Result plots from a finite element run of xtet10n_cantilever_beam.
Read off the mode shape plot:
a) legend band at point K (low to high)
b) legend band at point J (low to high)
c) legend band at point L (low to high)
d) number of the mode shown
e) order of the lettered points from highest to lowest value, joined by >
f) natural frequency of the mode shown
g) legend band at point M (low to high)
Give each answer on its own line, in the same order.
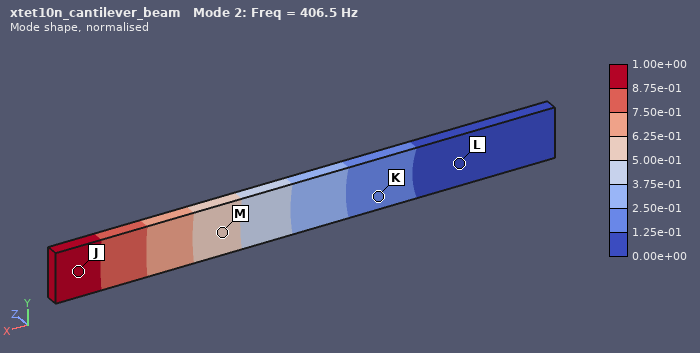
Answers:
1.25e-01 to 2.50e-01
8.75e-01 to 1.00e+00
0.00e+00 to 1.25e-01
2
J > M > K > L
406.5 Hz
5.00e-01 to 6.25e-01
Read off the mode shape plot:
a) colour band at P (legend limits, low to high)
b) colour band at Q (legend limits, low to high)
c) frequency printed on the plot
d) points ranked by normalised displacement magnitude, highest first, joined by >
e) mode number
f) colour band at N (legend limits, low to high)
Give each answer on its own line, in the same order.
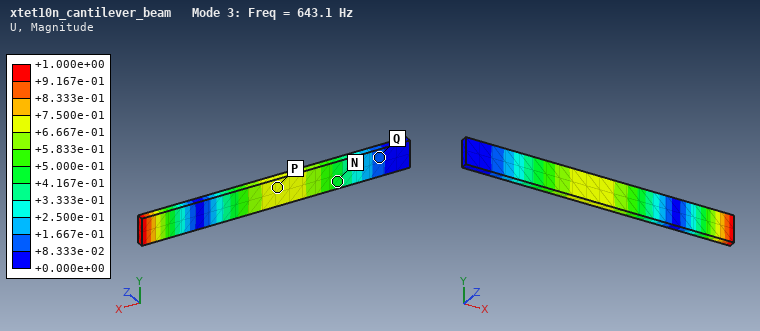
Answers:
+6.667e-01 to +7.500e-01
+8.333e-02 to +1.667e-01
643.1 Hz
P > N > Q
3
+4.167e-01 to +5.000e-01
